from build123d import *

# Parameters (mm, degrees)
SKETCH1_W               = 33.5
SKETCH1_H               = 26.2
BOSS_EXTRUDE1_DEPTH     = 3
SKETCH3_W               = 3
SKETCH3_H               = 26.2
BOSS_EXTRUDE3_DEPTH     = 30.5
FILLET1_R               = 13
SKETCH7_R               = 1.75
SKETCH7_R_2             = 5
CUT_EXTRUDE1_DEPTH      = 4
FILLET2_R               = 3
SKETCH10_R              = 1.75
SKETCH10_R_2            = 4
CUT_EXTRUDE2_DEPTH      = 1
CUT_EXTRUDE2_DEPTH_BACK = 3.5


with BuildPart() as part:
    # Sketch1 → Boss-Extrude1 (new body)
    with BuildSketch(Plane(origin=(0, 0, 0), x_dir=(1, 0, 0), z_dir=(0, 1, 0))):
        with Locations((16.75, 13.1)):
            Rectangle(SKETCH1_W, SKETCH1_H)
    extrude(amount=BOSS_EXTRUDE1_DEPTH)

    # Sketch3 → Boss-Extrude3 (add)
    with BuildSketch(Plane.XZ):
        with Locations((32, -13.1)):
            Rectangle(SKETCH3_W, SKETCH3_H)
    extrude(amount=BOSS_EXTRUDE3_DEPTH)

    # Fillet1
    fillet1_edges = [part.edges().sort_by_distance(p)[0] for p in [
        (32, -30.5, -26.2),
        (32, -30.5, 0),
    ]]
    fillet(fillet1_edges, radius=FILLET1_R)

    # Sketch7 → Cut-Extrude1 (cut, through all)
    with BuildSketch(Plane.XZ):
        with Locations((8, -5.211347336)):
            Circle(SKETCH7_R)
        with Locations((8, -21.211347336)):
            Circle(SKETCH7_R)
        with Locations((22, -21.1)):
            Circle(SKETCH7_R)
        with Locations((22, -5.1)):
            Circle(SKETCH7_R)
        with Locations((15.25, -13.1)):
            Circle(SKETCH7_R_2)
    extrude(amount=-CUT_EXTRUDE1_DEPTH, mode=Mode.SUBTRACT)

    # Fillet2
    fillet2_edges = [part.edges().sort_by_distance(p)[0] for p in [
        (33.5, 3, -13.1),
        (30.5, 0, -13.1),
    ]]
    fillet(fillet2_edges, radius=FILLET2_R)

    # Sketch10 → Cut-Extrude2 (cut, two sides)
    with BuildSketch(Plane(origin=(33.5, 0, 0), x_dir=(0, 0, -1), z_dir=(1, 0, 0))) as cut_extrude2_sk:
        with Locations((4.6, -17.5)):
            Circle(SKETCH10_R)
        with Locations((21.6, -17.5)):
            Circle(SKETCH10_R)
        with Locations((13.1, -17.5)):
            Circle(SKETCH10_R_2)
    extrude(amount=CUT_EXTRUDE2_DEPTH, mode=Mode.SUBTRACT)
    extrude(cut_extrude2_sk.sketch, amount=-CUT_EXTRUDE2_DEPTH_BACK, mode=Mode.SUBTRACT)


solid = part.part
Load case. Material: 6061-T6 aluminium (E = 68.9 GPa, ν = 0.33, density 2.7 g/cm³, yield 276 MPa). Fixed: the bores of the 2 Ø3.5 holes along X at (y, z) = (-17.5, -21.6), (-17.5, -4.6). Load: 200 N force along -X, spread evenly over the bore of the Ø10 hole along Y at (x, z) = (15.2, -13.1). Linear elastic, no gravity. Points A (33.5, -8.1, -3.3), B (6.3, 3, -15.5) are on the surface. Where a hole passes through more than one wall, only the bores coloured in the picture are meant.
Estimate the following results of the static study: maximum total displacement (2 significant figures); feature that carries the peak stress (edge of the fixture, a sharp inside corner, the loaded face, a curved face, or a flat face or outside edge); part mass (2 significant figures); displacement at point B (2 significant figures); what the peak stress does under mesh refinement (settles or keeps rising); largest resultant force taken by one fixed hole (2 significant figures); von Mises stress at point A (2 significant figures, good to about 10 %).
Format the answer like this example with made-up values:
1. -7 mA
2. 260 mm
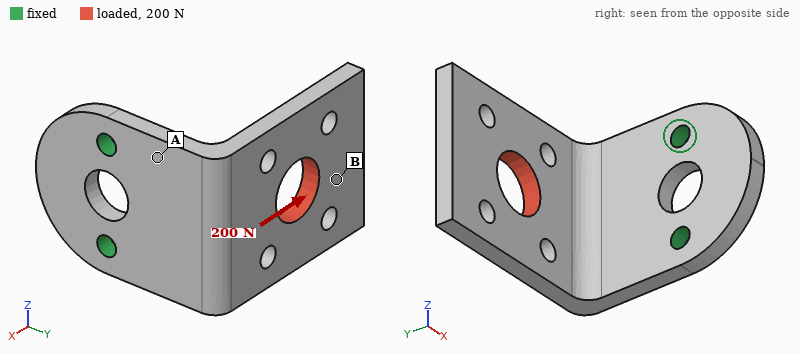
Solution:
1. 0.32 mm
2. edge of the fixture
3. 11 g
4. 0.27 mm
5. keeps rising
6. 100 N
7. 52 MPa
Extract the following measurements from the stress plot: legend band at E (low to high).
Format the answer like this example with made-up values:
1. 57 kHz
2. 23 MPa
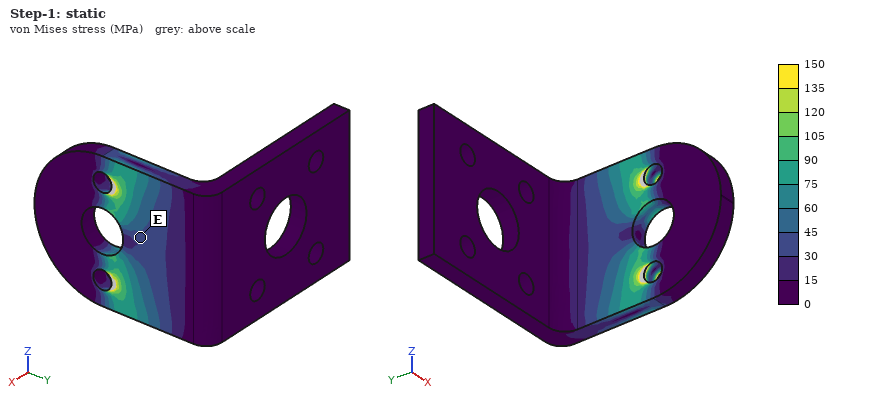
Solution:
1. 30 to 45 MPa
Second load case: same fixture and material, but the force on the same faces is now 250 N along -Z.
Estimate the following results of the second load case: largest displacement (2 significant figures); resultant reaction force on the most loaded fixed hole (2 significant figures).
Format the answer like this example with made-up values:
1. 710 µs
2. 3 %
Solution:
1. 0.23 mm
2. 340 N
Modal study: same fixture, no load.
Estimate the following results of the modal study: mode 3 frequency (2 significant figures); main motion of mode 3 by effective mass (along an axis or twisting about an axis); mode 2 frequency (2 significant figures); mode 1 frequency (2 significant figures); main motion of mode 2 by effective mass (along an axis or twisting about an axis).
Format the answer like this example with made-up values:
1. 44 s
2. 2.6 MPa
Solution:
1. 4000 Hz
2. along X
3. 2600 Hz
4. 1300 Hz
5. along Z
